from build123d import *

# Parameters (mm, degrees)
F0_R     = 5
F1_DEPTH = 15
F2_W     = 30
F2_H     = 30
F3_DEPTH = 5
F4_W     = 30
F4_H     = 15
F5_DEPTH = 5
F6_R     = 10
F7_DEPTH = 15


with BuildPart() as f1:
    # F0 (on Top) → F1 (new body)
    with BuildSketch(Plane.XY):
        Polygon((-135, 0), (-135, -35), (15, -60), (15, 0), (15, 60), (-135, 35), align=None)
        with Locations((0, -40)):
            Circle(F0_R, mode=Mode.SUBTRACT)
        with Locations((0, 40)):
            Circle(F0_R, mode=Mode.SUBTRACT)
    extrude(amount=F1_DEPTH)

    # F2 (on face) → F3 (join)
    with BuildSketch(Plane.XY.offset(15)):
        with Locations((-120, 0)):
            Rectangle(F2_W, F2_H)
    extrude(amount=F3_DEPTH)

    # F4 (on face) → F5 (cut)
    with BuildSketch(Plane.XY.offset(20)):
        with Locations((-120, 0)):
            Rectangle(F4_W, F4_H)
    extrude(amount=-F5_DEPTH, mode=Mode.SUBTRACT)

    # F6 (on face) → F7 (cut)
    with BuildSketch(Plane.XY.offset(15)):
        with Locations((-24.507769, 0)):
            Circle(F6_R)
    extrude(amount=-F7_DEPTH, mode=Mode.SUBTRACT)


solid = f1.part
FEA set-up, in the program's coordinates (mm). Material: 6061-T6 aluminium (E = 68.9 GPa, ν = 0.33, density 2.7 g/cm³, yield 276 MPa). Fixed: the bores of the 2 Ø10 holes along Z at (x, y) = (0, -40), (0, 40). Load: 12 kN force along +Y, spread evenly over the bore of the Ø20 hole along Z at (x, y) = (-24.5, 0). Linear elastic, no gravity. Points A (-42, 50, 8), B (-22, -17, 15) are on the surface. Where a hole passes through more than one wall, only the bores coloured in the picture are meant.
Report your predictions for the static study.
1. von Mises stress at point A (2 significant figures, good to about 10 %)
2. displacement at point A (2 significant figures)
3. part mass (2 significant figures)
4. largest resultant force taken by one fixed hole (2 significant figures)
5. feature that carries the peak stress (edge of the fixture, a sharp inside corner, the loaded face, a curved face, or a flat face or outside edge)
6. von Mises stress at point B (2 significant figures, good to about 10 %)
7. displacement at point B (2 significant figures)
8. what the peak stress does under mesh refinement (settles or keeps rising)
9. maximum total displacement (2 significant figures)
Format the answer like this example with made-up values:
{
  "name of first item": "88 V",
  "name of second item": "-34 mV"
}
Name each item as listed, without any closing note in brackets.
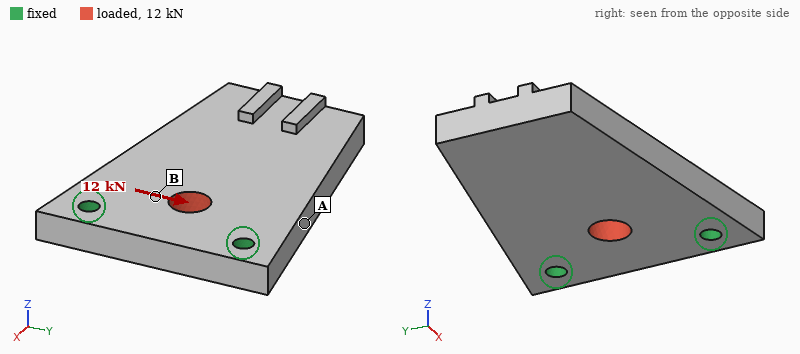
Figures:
{
  "von Mises stress at point A": "4.8 MPa",
  "displacement at point A": "12 µm",
  "part mass": "560 g",
  "largest resultant force taken by one fixed hole": "6.8 kN",
  "feature that carries the peak stress": "edge of the fixture",
  "von Mises stress at point B": "17 MPa",
  "displacement at point B": "9.5 µm",
  "what the peak stress does under mesh refinement": "keeps rising",
  "maximum total displacement": "15 µm"
}
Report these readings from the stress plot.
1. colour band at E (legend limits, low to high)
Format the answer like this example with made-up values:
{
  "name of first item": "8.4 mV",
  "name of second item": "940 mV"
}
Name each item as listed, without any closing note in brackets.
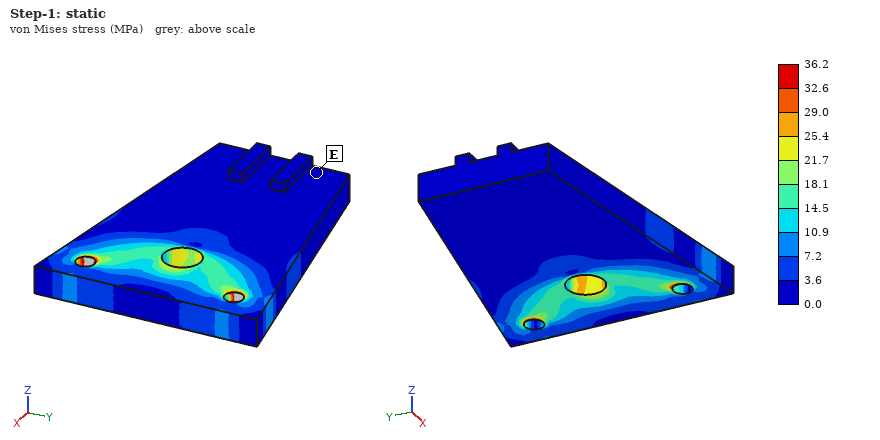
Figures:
{
  "colour band at E": "0.0 to 3.6 MPa"
}
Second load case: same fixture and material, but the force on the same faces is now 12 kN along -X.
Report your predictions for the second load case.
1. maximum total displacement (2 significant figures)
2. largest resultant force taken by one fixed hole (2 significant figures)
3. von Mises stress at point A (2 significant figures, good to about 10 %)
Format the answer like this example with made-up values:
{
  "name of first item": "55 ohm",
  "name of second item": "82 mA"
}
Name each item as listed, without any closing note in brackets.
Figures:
{
  "maximum total displacement": "13 µm",
  "largest resultant force taken by one fixed hole": "6.3 kN",
  "von Mises stress at point A": "7.1 MPa"
}
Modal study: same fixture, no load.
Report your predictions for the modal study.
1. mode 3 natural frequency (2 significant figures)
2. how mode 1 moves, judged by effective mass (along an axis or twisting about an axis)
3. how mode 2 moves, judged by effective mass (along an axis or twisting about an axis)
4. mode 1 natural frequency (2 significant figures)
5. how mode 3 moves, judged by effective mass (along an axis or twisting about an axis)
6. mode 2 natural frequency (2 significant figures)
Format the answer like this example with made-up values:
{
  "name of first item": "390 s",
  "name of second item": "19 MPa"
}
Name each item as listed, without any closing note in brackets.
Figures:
{
  "mode 3 natural frequency": "3700 Hz",
  "how mode 1 moves, judged by effective mass": "along Z",
  "how mode 2 moves, judged by effective mass": "twisting about X",
  "mode 1 natural frequency": "680 Hz",
  "how mode 3 moves, judged by effective mass": "along Y",
  "mode 2 natural frequency": "2600 Hz"
}
